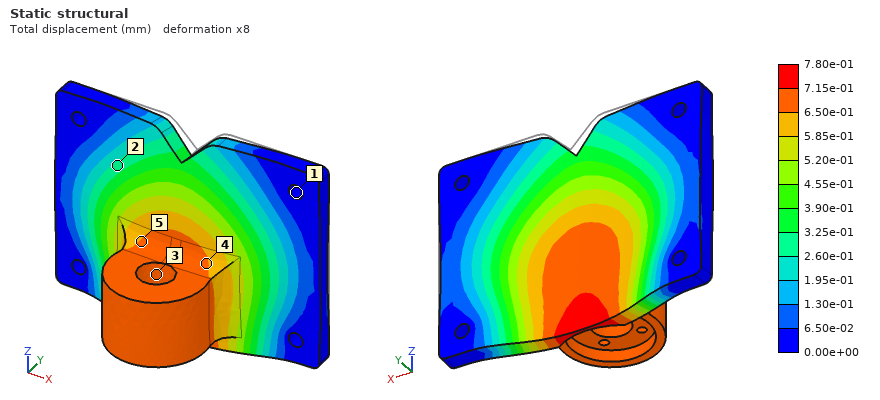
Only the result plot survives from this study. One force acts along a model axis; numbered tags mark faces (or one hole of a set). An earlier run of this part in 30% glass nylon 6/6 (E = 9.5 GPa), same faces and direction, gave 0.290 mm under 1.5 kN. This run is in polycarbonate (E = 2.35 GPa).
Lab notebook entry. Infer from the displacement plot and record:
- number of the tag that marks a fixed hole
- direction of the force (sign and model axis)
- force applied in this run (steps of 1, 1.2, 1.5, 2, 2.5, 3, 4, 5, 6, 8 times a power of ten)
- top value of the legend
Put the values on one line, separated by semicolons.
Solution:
1; -Y; 1 kN; 7.80e-01 mm
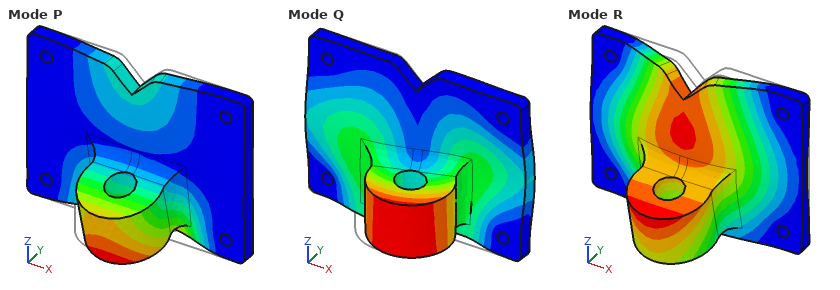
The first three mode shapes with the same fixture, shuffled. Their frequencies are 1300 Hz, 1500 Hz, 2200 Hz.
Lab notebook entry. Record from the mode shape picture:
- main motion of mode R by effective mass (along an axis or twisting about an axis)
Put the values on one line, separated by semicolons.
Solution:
along Y
